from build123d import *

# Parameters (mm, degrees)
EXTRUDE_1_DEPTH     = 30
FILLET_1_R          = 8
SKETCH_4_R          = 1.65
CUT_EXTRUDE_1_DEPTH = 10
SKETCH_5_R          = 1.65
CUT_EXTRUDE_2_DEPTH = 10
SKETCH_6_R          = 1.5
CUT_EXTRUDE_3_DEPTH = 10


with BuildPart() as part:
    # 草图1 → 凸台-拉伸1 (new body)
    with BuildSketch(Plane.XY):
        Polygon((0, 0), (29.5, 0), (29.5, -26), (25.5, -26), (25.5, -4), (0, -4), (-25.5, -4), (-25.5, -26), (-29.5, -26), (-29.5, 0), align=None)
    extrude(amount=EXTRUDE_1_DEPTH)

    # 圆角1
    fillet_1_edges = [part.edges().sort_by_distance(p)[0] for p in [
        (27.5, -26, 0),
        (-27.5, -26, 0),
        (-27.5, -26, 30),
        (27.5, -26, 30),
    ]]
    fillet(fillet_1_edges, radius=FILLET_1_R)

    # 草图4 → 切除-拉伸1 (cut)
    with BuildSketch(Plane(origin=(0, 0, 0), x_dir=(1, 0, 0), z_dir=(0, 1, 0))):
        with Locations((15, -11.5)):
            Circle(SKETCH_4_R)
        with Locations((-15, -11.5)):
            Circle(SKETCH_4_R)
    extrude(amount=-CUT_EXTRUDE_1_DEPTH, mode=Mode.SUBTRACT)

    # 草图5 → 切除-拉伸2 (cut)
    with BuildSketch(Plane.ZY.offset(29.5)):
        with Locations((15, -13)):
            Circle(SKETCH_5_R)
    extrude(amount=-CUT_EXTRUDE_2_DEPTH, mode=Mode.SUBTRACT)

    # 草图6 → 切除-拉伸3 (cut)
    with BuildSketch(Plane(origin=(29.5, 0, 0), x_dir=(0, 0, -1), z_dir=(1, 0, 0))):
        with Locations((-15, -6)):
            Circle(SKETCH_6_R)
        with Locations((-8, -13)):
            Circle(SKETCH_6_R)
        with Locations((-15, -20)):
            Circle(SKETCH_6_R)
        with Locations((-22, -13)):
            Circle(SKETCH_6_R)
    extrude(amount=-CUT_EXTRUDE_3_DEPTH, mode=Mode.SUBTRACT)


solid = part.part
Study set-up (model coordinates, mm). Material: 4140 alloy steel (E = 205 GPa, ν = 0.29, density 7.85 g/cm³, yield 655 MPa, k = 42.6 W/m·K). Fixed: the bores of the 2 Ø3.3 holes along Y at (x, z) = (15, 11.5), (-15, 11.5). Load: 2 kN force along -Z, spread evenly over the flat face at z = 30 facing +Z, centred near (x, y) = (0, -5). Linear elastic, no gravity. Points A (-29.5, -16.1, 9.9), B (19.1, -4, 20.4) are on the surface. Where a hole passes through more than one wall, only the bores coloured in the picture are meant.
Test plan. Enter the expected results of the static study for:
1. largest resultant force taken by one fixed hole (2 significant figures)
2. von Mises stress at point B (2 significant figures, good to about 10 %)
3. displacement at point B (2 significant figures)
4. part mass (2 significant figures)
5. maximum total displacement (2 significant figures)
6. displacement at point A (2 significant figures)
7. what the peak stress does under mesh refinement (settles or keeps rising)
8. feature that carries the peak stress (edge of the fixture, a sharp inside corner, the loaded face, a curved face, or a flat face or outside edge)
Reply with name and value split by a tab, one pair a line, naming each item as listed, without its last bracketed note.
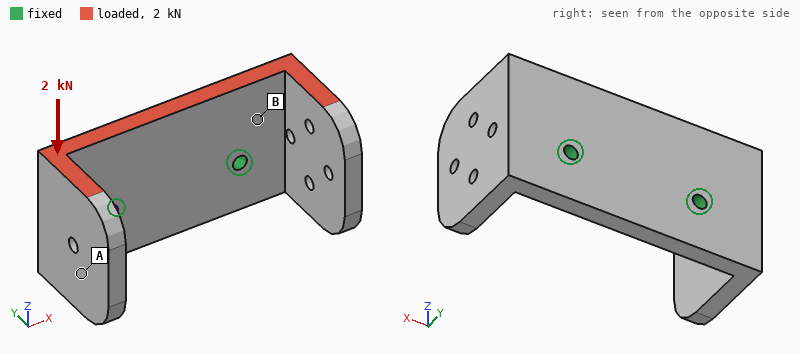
largest resultant force taken by one fixed hole	1.0 kN
von Mises stress at point B	23 MPa
displacement at point B	4.9 µm
part mass	94 g
maximum total displacement	23 µm
displacement at point A	13 µm
what the peak stress does under mesh refinement	keeps rising
feature that carries the peak stress	edge of the fixture
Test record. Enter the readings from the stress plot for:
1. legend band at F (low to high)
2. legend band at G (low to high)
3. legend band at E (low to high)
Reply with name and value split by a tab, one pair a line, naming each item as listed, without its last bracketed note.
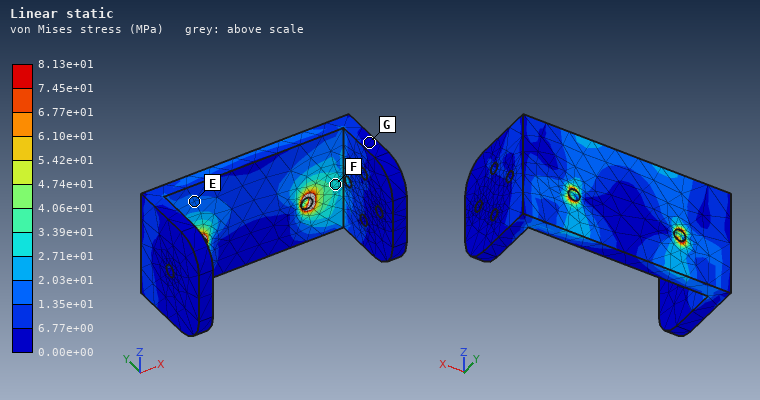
legend band at F	2.71e+01 to 3.39e+01 MPa
legend band at G	0.00e+00 to 6.77e+00 MPa
legend band at E	1.35e+01 to 2.03e+01 MPa
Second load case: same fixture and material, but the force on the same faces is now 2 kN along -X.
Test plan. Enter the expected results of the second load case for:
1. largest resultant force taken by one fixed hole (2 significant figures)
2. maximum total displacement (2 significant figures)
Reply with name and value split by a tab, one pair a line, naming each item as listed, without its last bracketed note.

largest resultant force taken by one fixed hole	1.5 kN
maximum total displacement	48 µm
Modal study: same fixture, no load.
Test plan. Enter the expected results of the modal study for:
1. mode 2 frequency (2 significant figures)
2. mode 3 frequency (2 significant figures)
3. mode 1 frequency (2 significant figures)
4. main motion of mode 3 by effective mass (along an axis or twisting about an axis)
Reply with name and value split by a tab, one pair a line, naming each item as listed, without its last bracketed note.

mode 2 frequency	3100 Hz
mode 3 frequency	3800 Hz
mode 1 frequency	3000 Hz
main motion of mode 3 by effective mass	along Z
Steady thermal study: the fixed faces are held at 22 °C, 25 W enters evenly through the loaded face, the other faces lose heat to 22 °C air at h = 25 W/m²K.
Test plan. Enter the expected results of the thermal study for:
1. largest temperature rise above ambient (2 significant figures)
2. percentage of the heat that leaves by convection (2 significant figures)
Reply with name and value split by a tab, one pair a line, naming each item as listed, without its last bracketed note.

largest temperature rise above ambient	47 K
percentage of the heat that leaves by convection	17 %
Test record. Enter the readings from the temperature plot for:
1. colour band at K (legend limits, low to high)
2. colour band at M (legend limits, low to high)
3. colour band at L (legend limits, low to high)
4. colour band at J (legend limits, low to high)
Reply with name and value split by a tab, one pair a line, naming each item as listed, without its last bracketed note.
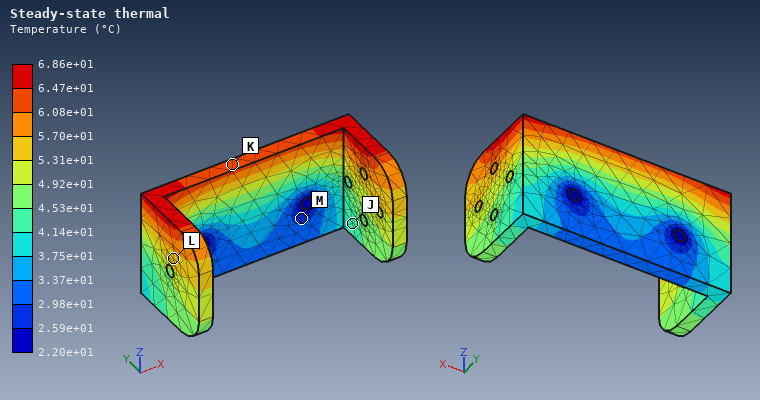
colour band at K	6.08e+01 to 6.47e+01 °C
colour band at M	2.59e+01 to 2.98e+01 °C
colour band at L	5.31e+01 to 5.70e+01 °C
colour band at J	4.14e+01 to 4.53e+01 °C
